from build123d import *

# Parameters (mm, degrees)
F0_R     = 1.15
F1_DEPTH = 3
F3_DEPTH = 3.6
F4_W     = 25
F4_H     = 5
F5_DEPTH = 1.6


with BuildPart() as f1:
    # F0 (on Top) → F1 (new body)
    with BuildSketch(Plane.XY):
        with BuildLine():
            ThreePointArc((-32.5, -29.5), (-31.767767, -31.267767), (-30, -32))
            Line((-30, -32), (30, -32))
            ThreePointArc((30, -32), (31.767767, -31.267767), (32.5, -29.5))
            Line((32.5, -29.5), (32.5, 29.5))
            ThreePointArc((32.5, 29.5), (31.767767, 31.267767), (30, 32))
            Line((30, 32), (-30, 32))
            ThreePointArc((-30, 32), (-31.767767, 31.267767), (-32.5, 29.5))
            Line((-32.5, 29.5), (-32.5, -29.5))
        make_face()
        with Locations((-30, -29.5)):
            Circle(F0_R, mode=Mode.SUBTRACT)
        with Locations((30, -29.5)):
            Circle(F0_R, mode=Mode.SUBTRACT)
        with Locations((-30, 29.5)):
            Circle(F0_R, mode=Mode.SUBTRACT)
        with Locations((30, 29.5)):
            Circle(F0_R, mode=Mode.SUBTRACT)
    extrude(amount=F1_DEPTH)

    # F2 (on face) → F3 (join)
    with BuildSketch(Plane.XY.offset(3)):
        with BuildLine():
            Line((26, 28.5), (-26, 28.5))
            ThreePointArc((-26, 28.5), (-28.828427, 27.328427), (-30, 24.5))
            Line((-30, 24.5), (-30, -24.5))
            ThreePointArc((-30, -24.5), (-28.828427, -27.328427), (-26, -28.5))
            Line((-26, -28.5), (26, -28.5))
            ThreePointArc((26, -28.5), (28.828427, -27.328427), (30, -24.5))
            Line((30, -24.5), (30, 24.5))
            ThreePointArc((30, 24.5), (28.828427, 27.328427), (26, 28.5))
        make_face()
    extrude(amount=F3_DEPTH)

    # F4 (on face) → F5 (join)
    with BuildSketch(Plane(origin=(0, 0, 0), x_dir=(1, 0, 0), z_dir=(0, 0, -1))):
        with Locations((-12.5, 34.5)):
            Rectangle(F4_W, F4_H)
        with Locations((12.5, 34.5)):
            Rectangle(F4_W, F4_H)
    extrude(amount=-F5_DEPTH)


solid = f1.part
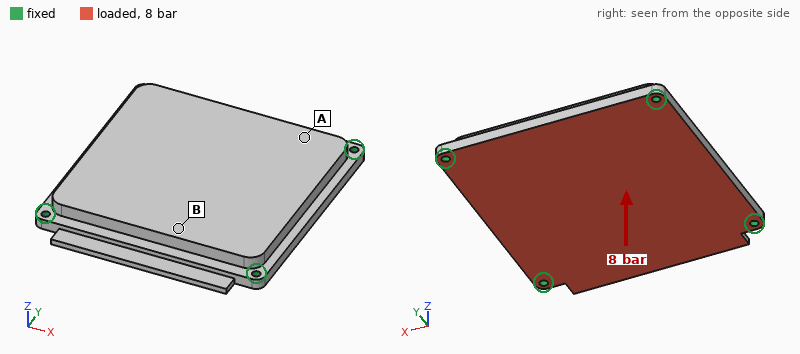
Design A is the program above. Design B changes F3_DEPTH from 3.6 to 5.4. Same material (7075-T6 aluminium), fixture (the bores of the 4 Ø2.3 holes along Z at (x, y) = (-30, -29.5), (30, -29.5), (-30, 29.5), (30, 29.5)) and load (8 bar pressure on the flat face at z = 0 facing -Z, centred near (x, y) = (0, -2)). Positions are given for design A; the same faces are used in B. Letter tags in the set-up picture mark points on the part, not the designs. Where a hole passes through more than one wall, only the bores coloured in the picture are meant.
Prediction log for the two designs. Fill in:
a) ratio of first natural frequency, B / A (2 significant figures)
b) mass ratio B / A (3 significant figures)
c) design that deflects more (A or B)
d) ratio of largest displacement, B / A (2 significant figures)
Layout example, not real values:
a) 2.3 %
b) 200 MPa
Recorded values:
a) 1.2
b) 1.24
c) A
d) 0.63
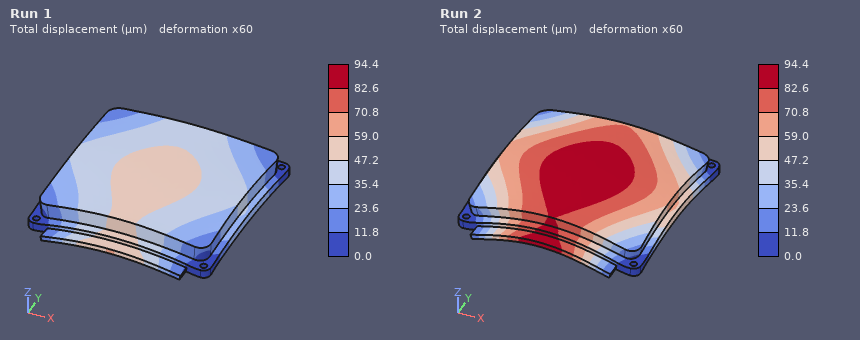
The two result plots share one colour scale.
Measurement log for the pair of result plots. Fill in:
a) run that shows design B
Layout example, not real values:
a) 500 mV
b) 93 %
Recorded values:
a) Run 1
